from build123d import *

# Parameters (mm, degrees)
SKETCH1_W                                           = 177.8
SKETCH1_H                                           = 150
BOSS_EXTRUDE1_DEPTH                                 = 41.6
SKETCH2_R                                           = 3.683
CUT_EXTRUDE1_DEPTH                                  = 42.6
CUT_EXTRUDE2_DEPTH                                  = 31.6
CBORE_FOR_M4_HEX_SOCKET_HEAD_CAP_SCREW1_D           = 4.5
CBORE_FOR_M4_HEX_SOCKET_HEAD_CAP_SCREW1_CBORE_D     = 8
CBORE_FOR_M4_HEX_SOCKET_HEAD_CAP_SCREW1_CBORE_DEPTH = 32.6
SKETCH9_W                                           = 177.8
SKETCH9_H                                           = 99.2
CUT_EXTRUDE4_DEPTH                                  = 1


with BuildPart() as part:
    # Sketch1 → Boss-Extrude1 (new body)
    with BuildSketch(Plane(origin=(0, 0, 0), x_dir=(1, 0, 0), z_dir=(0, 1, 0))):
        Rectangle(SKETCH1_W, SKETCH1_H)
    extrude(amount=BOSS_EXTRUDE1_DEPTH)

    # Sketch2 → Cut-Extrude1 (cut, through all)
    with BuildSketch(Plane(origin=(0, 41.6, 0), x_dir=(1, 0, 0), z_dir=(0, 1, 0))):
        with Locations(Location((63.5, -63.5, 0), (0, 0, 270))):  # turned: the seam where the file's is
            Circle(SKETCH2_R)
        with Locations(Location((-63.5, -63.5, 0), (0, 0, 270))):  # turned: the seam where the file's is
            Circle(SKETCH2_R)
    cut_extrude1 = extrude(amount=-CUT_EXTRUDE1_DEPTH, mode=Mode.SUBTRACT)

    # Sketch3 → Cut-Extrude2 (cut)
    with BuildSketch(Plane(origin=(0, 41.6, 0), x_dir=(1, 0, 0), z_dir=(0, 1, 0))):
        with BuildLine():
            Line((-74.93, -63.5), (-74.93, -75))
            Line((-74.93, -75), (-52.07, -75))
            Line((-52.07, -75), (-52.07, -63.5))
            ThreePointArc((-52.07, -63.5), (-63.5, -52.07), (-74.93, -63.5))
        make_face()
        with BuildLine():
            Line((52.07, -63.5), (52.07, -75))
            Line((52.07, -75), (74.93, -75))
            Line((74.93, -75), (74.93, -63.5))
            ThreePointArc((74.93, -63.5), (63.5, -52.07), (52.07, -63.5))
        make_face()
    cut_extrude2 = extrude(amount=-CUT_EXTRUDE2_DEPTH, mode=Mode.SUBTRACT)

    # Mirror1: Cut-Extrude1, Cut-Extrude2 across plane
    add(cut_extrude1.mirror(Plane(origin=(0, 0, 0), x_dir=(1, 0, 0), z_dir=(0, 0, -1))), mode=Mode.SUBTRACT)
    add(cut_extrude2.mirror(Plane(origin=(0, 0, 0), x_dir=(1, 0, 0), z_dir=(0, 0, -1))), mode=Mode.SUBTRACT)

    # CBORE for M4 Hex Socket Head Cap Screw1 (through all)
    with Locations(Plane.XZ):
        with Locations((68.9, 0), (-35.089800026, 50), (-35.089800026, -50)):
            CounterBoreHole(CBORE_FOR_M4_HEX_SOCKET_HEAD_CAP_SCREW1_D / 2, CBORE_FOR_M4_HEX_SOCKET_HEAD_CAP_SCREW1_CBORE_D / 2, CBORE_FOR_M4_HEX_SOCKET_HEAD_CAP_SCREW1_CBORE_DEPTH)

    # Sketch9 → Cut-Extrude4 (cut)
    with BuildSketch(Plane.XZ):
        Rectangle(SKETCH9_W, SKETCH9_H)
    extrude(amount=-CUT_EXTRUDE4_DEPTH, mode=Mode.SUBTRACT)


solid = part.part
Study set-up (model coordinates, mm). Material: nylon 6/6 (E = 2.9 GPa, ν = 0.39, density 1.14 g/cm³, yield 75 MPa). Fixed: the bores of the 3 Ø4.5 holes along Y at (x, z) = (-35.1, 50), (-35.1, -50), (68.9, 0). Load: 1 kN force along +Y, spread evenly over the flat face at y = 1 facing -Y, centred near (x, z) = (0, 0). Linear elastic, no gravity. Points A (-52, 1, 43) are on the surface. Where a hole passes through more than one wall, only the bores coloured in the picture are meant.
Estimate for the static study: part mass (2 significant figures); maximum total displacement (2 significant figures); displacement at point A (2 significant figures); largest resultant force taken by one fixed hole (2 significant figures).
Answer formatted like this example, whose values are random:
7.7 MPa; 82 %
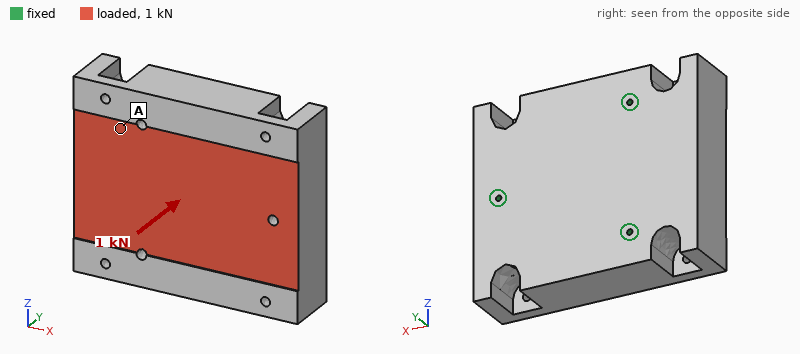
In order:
1.2 kg; 23 µm; 14 µm; 340 N
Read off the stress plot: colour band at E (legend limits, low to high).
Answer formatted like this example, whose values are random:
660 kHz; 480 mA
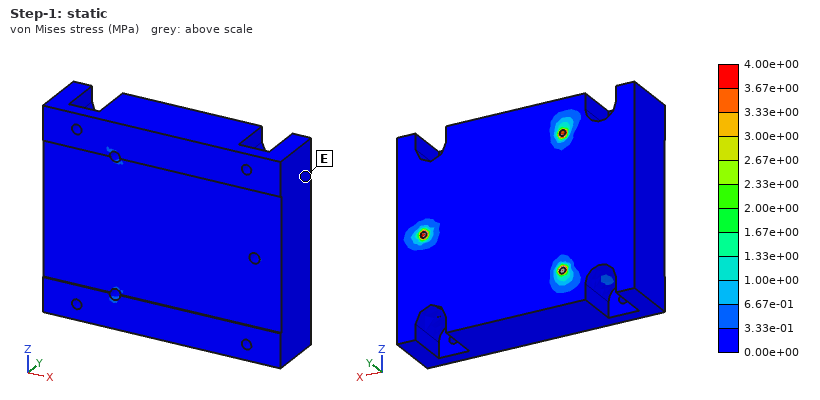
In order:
0.00e+00 to 3.33e-01 MPa
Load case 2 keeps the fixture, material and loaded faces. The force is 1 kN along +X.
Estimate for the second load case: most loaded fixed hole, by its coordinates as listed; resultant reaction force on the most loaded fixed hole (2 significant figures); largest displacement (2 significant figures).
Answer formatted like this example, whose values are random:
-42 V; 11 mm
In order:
(68.9, 0); 520 N; 39 µm
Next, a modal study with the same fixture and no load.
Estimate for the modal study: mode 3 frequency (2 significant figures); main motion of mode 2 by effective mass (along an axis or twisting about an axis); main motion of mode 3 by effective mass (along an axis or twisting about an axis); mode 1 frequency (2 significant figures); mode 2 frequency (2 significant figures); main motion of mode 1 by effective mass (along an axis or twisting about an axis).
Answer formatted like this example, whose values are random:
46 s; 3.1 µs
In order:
1300 Hz; along X; along Y; 920 Hz; 990 Hz; along Z
